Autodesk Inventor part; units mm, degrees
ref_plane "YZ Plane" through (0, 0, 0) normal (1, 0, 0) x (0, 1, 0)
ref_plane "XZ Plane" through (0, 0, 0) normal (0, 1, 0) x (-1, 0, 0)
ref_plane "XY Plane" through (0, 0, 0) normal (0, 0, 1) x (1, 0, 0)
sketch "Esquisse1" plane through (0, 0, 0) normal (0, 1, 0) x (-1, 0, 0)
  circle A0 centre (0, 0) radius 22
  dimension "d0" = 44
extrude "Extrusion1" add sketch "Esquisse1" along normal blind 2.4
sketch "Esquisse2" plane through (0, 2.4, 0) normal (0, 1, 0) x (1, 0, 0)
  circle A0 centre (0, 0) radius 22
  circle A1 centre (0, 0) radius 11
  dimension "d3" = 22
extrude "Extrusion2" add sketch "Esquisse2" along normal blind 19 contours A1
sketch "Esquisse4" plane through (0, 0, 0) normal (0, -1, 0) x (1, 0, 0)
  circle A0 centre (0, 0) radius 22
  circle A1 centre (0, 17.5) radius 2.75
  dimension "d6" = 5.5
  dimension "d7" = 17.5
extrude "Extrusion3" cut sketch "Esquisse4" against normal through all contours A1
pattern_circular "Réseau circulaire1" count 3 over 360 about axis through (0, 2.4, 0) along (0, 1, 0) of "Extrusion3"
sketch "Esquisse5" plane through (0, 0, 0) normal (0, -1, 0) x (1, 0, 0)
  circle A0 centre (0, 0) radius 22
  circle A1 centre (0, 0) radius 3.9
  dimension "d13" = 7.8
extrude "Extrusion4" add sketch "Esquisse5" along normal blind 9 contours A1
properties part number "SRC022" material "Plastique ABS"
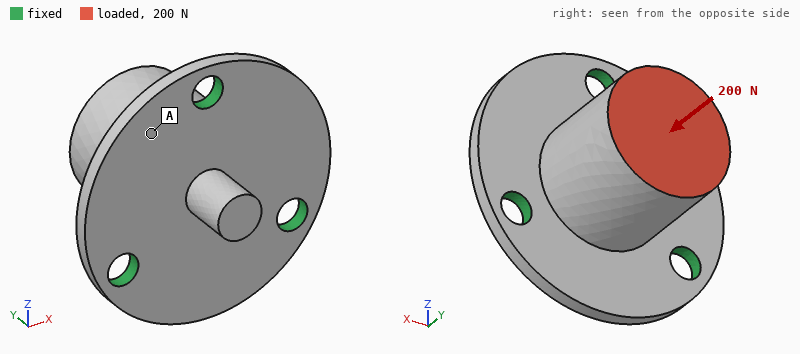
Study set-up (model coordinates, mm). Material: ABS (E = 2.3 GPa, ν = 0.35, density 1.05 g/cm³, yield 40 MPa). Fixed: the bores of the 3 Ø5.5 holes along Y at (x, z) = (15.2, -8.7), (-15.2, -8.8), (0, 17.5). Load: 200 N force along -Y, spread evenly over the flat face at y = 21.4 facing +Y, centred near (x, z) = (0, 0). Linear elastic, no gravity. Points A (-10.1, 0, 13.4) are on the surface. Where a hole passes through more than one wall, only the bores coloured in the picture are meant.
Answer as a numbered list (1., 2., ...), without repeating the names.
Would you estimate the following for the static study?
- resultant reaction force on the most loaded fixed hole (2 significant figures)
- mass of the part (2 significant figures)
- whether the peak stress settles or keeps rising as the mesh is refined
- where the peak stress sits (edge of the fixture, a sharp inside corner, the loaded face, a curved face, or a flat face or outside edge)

1. 72 N
2. 12 g
3. keeps rising
4. edge of the fixture
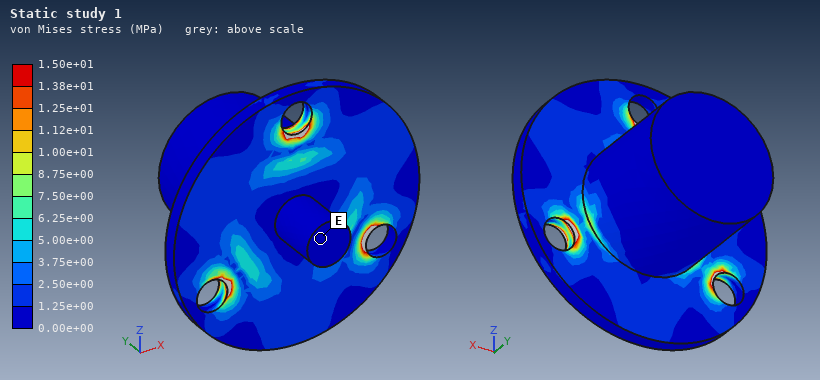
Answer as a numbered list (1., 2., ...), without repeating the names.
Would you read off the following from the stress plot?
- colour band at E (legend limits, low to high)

1. 0.00e+00 to 1.25e+00 MPa
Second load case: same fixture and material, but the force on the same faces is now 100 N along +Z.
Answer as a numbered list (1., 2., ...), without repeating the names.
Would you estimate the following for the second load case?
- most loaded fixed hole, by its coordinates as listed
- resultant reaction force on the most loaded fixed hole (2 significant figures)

1. (0, 17.5)
2. 110 N
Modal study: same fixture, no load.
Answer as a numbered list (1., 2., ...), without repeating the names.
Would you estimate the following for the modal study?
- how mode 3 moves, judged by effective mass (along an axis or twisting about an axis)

1. along Y
